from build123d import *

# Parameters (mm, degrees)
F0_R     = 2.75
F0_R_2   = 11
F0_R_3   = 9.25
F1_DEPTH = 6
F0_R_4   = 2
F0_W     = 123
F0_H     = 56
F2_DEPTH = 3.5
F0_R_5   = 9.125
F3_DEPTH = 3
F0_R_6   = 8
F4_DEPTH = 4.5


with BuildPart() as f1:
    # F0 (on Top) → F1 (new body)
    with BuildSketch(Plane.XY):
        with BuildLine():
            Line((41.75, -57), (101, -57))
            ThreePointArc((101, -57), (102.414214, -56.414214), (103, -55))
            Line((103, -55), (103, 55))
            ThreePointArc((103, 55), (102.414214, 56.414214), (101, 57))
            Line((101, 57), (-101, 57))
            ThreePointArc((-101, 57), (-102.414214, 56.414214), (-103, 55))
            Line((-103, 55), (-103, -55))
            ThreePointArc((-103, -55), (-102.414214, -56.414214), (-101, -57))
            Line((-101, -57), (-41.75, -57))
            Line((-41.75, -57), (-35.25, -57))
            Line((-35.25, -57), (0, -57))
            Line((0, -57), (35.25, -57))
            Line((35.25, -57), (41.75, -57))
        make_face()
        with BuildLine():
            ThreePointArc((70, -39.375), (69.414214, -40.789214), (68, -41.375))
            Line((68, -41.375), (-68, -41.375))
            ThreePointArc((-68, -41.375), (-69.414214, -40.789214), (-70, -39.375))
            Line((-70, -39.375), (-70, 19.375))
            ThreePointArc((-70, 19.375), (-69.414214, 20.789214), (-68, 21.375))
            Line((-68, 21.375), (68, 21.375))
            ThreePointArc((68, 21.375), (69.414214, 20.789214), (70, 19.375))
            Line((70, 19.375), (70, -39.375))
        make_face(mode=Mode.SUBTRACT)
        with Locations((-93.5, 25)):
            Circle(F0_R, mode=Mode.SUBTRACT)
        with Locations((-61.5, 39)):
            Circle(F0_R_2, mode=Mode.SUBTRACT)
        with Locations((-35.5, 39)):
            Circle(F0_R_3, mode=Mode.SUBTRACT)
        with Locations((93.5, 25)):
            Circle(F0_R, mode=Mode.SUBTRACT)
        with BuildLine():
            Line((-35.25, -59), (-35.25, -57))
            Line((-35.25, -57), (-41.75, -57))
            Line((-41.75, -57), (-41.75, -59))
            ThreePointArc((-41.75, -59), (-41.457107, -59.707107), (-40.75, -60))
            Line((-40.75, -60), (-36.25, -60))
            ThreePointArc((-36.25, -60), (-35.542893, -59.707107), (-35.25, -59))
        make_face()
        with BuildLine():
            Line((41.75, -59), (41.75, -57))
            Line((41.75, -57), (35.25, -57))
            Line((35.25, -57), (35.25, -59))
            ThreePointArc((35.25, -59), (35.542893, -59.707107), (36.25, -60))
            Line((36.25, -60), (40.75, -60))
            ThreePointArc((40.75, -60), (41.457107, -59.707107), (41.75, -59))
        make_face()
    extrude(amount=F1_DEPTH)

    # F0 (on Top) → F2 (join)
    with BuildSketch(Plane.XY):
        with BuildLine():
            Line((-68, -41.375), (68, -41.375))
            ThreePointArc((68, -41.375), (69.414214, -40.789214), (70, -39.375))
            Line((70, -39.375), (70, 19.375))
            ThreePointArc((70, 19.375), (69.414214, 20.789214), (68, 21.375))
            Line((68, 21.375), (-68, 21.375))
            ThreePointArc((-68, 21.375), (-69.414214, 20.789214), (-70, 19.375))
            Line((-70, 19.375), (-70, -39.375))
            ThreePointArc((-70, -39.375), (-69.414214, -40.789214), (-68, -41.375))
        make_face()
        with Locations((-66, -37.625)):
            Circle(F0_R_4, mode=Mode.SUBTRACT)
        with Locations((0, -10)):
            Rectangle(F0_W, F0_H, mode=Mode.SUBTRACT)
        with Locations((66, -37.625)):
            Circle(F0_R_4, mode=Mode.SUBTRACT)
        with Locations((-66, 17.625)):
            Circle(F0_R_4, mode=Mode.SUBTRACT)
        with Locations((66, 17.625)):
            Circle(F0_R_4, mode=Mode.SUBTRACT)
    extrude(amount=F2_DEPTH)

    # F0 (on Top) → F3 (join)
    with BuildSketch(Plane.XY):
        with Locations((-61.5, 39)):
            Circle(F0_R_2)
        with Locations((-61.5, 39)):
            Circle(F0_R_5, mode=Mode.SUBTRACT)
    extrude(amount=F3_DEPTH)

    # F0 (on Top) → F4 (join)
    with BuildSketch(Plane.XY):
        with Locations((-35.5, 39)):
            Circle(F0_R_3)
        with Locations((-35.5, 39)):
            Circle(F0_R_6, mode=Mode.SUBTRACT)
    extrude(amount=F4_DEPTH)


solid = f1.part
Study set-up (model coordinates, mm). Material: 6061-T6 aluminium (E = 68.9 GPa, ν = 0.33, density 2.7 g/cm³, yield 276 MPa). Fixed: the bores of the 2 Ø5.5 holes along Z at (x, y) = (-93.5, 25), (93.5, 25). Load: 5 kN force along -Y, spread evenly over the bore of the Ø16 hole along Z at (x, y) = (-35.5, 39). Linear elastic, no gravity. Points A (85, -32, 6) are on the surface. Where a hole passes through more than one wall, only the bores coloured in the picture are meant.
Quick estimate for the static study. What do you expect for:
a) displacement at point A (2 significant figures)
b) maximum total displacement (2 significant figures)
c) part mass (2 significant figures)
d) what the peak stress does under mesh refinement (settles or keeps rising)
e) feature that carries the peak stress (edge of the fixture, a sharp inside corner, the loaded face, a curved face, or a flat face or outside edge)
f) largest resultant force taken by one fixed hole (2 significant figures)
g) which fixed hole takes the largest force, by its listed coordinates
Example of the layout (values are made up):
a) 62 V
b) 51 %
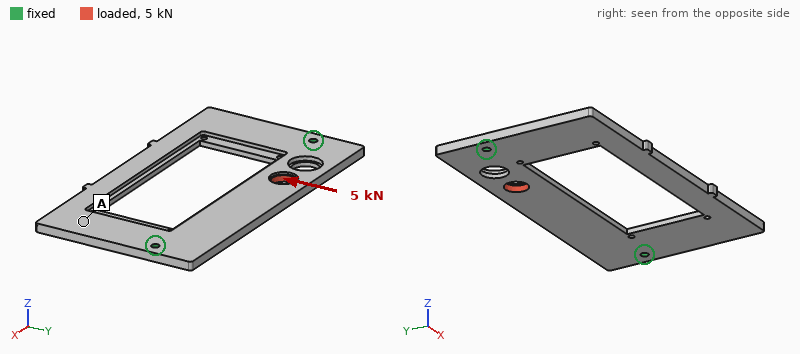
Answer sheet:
a) 0.045 mm
b) 0.16 mm
c) 250 g
d) keeps rising
e) a sharp inside corner
f) 3.7 kN
g) (-93.5, 25)
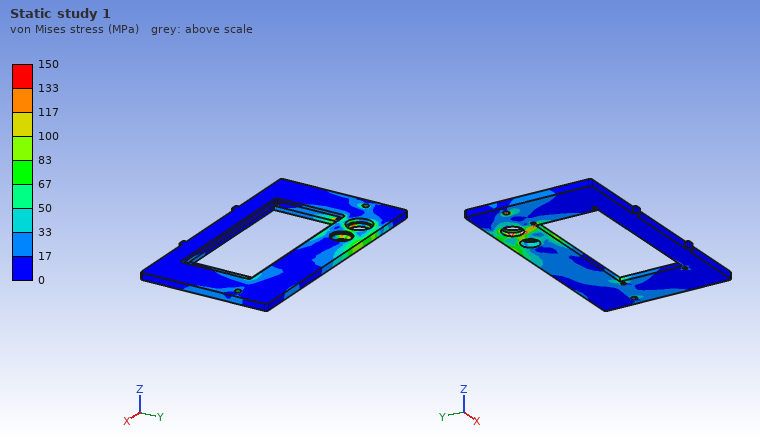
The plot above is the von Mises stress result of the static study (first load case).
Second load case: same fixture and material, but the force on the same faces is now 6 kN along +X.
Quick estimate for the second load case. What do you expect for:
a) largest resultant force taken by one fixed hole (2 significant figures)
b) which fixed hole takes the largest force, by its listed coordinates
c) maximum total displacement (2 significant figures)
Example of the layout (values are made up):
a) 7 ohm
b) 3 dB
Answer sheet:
a) 3.4 kN
b) (-93.5, 25)
c) 51 µm
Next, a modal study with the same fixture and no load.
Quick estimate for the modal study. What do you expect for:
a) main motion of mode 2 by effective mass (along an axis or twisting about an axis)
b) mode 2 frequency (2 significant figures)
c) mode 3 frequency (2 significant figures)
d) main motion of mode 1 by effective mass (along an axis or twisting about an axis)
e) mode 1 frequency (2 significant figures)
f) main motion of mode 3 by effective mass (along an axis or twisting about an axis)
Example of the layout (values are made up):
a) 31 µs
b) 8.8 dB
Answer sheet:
a) twisting about Y
b) 740 Hz
c) 840 Hz
d) along Z
e) 420 Hz
f) along Z
